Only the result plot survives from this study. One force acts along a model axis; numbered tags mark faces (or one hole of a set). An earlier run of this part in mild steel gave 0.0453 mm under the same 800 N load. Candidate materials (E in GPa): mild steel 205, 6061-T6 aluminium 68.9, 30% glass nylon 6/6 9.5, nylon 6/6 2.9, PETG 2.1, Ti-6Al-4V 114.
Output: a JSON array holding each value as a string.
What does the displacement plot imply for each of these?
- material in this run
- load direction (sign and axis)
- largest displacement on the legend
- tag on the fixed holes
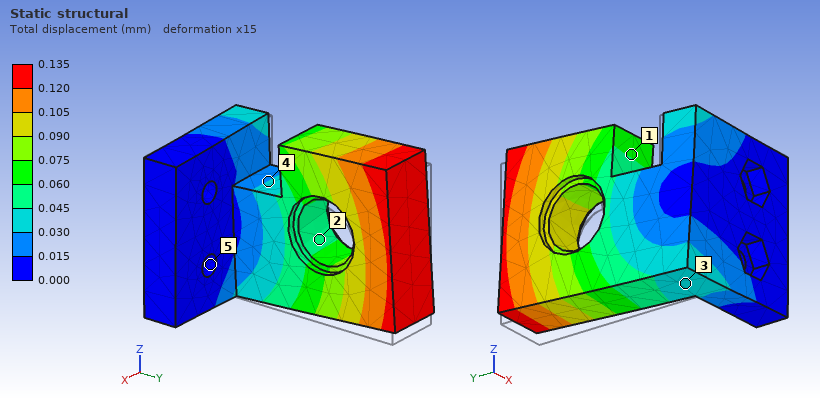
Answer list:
["6061-T6 aluminium", "+Z", "0.135 mm", "5"]
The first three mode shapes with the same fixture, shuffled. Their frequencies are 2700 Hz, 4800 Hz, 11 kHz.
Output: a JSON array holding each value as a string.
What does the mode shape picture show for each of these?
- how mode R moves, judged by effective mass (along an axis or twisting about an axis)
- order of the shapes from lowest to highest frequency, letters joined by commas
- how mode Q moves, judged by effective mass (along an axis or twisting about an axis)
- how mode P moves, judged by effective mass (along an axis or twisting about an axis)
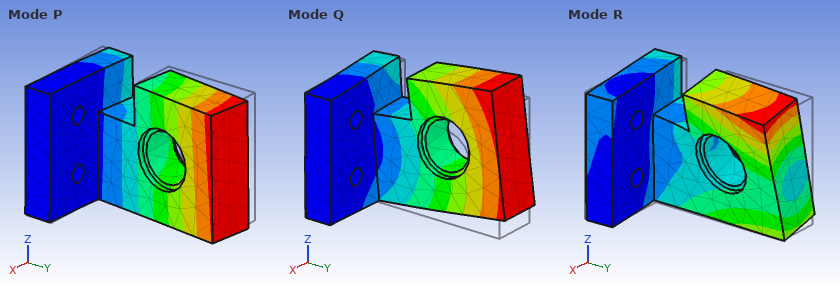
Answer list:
["along Y", "P, Q, R", "along Z", "along X"]
